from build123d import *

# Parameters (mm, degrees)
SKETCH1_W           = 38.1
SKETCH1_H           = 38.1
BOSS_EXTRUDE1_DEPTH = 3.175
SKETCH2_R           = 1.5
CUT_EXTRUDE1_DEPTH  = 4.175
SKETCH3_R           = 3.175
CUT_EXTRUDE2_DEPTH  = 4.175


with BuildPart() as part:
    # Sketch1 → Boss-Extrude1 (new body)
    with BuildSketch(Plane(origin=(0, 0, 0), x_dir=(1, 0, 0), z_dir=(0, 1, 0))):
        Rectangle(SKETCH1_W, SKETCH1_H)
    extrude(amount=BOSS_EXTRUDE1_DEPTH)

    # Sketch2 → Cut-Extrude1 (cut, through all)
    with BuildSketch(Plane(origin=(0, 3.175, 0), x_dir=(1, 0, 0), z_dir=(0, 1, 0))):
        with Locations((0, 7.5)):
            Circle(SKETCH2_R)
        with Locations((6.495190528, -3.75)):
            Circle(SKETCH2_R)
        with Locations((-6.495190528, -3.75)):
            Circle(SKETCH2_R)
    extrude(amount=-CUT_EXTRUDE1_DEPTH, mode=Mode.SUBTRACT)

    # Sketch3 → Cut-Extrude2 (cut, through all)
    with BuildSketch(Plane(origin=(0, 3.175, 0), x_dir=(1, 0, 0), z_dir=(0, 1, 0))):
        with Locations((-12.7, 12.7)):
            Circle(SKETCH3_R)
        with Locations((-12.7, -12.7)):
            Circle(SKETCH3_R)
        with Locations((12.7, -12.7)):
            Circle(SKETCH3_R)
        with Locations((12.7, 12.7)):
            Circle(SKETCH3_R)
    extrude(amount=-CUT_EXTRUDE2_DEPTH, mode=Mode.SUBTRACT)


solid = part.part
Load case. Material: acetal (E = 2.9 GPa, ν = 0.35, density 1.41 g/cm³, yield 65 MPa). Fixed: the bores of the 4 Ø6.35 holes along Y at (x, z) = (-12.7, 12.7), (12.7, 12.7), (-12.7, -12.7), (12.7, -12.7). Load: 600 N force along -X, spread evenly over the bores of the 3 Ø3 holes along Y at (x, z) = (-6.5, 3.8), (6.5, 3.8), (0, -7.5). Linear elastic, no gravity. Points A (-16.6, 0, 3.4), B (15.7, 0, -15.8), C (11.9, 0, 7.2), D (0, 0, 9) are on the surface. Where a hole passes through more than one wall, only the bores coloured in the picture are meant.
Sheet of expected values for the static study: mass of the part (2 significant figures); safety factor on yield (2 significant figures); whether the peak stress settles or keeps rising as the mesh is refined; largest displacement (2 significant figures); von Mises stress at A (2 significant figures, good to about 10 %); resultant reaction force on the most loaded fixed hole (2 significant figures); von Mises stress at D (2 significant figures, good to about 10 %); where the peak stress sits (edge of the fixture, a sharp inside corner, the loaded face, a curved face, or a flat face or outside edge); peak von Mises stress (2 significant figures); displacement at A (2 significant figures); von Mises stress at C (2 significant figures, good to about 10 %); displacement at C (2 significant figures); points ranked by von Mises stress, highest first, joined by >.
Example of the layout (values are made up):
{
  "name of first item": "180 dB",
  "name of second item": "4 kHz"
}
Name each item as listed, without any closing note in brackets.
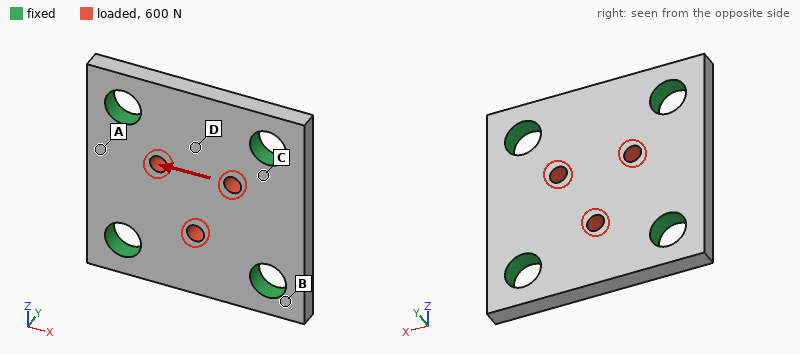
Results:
{
  "mass of the part": "5.8 g",
  "safety factor on yield": "5.1",
  "whether the peak stress settles or keeps rising as the mesh is refined": "settles",
  "largest displacement": "27 µm",
  "von Mises stress at A": "1.9 MPa",
  "resultant reaction force on the most loaded fixed hole": "160 N",
  "von Mises stress at D": "3.7 MPa",
  "where the peak stress sits": "the loaded face",
  "peak von Mises stress": "13 MPa",
  "displacement at A": "15 µm",
  "von Mises stress at C": "5.0 MPa",
  "displacement at C": "9.5 µm",
  "points ranked by von Mises stress, highest first, joined by >": "C > D > A > B"
}
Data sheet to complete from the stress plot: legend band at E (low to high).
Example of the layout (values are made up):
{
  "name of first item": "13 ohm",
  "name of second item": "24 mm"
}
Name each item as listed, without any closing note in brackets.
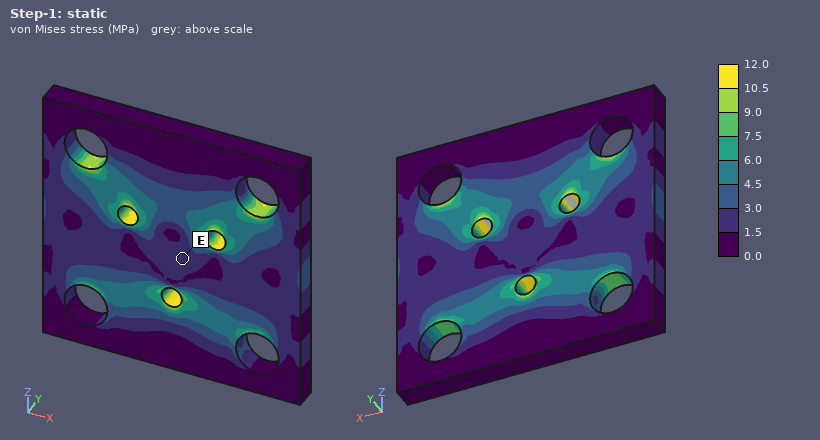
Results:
{
  "legend band at E": "1.5 to 3.0 MPa"
}
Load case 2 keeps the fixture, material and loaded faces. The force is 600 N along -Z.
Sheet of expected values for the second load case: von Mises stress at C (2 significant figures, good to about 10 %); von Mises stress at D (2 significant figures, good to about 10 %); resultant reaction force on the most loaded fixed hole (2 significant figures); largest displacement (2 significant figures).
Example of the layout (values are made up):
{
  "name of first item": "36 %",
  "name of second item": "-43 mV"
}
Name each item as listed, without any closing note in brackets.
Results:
{
  "von Mises stress at C": "3.8 MPa",
  "von Mises stress at D": "1.5 MPa",
  "resultant reaction force on the most loaded fixed hole": "170 N",
  "largest displacement": "27 µm"
}
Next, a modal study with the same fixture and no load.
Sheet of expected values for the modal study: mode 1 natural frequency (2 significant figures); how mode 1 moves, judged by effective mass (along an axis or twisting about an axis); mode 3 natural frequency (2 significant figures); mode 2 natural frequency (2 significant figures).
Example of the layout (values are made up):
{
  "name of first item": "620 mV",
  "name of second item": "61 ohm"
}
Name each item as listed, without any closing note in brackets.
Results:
{
  "mode 1 natural frequency": "6800 Hz",
  "how mode 1 moves, judged by effective mass": "along Y",
  "mode 3 natural frequency": "9600 Hz",
  "mode 2 natural frequency": "9600 Hz"
}
